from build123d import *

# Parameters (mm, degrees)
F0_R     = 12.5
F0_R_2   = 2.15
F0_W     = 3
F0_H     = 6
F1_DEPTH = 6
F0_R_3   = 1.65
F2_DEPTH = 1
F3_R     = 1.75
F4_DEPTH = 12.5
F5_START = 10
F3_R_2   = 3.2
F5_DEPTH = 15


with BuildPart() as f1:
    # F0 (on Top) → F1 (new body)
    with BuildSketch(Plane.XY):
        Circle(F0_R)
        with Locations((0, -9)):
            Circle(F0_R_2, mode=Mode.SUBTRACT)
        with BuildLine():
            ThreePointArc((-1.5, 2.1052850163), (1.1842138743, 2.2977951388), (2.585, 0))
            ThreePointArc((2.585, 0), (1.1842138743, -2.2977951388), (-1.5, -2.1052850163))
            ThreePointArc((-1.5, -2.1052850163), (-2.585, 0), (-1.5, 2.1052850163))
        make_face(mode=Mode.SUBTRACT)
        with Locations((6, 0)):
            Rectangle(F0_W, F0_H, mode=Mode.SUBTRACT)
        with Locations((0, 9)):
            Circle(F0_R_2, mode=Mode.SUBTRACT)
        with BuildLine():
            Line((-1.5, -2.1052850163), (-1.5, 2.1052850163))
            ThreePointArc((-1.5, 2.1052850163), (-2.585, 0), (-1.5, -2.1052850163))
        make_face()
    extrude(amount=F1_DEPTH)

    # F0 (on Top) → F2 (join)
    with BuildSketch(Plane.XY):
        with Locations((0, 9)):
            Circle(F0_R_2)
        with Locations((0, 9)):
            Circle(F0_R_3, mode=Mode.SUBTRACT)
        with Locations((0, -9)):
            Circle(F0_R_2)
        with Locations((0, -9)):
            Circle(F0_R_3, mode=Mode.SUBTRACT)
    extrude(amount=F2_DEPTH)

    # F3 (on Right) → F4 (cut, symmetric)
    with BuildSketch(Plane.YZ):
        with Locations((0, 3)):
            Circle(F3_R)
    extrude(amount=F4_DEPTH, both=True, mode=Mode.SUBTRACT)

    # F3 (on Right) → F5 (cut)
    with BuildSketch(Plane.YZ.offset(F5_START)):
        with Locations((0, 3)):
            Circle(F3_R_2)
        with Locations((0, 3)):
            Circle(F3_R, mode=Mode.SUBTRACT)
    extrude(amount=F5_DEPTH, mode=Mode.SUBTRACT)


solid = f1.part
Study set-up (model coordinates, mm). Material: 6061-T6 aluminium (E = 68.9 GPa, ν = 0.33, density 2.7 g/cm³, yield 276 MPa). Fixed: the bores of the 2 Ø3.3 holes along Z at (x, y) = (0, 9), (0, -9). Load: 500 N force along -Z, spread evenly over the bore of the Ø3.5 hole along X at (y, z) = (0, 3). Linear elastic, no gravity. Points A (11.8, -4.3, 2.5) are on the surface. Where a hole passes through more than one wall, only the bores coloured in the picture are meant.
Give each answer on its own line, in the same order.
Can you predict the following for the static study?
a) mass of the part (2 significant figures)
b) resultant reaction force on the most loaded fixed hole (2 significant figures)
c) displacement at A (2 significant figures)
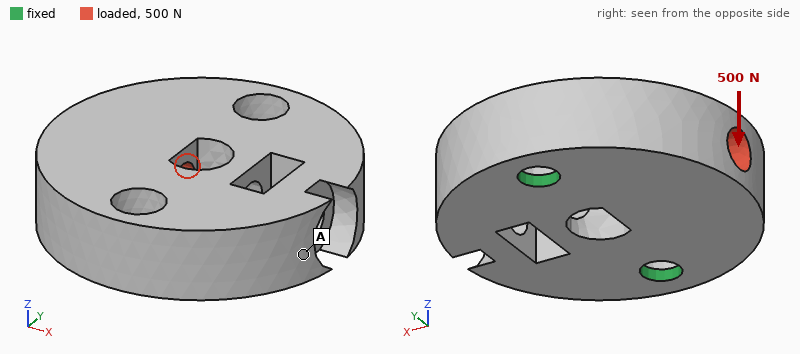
6.3 g
290 N
42 µm
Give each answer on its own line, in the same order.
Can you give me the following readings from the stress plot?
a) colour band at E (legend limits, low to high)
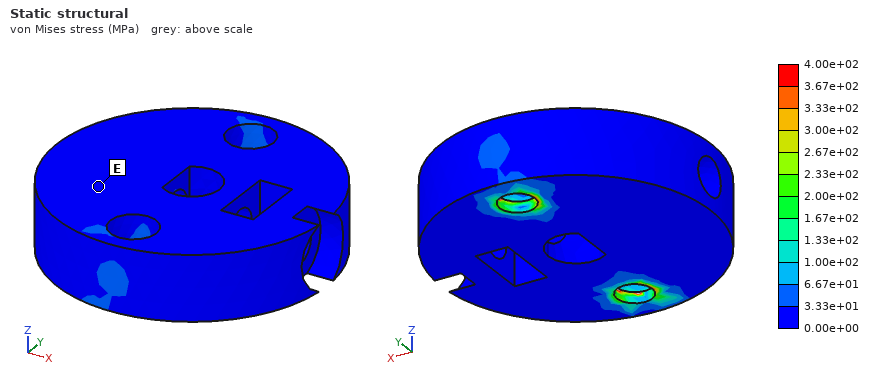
0.00e+00 to 3.33e+01 MPa
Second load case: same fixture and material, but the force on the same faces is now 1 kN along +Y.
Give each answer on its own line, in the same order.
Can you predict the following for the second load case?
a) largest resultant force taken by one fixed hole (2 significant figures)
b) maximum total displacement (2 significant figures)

620 N
7.8 µm
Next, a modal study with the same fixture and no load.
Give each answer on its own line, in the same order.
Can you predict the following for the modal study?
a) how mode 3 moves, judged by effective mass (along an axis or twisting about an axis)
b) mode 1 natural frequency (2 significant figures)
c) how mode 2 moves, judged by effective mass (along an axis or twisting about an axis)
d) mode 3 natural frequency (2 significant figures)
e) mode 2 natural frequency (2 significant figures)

twisting about Z
8500 Hz
along Z
28 kHz
26 kHz
